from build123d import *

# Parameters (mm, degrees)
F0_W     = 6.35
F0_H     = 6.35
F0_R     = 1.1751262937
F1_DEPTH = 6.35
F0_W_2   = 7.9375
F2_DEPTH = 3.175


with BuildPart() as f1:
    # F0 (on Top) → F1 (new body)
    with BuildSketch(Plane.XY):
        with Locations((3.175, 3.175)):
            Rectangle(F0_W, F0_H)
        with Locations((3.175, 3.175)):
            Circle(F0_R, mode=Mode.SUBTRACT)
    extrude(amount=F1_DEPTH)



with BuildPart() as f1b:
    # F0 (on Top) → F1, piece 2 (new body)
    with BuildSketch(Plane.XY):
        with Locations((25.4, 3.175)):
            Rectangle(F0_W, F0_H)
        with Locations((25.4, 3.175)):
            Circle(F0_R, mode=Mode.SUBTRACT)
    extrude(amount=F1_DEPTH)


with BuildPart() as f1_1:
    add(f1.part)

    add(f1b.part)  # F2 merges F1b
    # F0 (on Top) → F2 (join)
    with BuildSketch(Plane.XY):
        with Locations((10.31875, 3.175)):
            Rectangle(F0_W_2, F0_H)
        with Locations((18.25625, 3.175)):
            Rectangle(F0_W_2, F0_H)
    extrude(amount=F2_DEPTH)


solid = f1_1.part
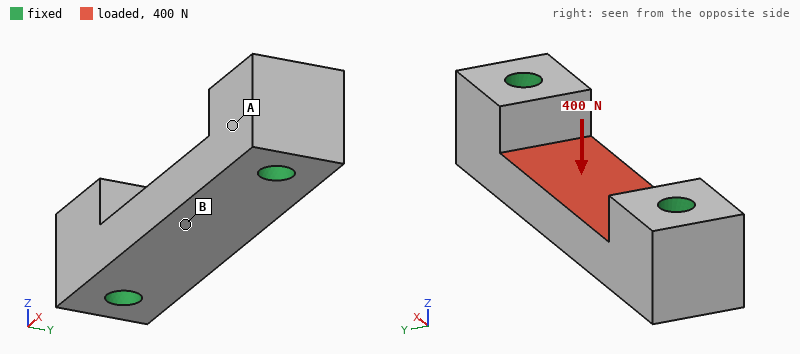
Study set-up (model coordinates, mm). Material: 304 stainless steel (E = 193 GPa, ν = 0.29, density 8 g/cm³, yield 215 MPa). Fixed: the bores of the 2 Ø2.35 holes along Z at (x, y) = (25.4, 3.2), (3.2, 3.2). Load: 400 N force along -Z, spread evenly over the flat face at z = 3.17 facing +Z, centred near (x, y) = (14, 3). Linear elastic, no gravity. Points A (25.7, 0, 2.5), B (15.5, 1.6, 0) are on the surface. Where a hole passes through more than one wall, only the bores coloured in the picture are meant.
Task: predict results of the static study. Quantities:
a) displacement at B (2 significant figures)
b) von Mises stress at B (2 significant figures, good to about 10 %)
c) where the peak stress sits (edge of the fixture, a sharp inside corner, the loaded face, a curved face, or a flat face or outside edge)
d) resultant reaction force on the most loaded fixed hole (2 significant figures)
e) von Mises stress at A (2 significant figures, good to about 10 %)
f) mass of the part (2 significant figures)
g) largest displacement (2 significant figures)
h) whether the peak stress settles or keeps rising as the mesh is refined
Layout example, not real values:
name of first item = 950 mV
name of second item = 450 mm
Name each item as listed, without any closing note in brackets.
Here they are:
displacement at B = 3.2 µm
von Mises stress at B = 35 MPa
where the peak stress sits = edge of the fixture
resultant reaction force on the most loaded fixed hole = 200 N
von Mises stress at A = 6.4 MPa
mass of the part = 6.2 g
largest displacement = 3.4 µm
whether the peak stress settles or keeps rising as the mesh is refined = keeps rising
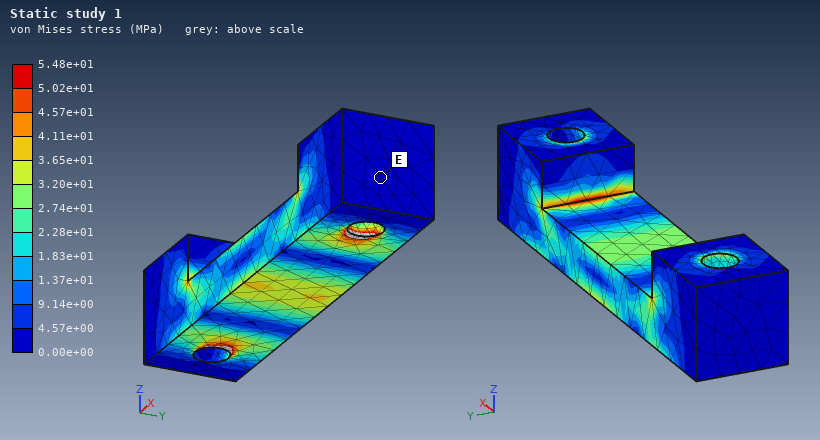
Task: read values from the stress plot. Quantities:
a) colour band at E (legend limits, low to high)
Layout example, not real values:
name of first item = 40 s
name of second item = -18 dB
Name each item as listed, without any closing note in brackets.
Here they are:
colour band at E = 0.00e+00 to 4.57e+00 MPa
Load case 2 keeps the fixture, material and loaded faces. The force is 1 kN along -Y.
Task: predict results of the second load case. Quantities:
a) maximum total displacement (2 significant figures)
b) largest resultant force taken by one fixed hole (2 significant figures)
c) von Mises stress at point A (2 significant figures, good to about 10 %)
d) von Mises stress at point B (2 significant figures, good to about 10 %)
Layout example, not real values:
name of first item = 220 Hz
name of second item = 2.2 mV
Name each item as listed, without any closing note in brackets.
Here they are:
maximum total displacement = 8.1 µm
largest resultant force taken by one fixed hole = 500 N
von Mises stress at point A = 25 MPa
von Mises stress at point B = 40 MPa
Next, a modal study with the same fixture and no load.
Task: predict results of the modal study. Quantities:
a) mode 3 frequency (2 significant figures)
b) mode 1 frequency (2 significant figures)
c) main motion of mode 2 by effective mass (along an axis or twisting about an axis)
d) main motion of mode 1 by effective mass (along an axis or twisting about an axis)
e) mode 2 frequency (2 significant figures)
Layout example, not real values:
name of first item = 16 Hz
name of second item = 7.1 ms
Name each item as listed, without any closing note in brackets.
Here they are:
mode 3 frequency = 65 kHz
mode 1 frequency = 39 kHz
main motion of mode 2 by effective mass = along Y
main motion of mode 1 by effective mass = along Z
mode 2 frequency = 45 kHz
